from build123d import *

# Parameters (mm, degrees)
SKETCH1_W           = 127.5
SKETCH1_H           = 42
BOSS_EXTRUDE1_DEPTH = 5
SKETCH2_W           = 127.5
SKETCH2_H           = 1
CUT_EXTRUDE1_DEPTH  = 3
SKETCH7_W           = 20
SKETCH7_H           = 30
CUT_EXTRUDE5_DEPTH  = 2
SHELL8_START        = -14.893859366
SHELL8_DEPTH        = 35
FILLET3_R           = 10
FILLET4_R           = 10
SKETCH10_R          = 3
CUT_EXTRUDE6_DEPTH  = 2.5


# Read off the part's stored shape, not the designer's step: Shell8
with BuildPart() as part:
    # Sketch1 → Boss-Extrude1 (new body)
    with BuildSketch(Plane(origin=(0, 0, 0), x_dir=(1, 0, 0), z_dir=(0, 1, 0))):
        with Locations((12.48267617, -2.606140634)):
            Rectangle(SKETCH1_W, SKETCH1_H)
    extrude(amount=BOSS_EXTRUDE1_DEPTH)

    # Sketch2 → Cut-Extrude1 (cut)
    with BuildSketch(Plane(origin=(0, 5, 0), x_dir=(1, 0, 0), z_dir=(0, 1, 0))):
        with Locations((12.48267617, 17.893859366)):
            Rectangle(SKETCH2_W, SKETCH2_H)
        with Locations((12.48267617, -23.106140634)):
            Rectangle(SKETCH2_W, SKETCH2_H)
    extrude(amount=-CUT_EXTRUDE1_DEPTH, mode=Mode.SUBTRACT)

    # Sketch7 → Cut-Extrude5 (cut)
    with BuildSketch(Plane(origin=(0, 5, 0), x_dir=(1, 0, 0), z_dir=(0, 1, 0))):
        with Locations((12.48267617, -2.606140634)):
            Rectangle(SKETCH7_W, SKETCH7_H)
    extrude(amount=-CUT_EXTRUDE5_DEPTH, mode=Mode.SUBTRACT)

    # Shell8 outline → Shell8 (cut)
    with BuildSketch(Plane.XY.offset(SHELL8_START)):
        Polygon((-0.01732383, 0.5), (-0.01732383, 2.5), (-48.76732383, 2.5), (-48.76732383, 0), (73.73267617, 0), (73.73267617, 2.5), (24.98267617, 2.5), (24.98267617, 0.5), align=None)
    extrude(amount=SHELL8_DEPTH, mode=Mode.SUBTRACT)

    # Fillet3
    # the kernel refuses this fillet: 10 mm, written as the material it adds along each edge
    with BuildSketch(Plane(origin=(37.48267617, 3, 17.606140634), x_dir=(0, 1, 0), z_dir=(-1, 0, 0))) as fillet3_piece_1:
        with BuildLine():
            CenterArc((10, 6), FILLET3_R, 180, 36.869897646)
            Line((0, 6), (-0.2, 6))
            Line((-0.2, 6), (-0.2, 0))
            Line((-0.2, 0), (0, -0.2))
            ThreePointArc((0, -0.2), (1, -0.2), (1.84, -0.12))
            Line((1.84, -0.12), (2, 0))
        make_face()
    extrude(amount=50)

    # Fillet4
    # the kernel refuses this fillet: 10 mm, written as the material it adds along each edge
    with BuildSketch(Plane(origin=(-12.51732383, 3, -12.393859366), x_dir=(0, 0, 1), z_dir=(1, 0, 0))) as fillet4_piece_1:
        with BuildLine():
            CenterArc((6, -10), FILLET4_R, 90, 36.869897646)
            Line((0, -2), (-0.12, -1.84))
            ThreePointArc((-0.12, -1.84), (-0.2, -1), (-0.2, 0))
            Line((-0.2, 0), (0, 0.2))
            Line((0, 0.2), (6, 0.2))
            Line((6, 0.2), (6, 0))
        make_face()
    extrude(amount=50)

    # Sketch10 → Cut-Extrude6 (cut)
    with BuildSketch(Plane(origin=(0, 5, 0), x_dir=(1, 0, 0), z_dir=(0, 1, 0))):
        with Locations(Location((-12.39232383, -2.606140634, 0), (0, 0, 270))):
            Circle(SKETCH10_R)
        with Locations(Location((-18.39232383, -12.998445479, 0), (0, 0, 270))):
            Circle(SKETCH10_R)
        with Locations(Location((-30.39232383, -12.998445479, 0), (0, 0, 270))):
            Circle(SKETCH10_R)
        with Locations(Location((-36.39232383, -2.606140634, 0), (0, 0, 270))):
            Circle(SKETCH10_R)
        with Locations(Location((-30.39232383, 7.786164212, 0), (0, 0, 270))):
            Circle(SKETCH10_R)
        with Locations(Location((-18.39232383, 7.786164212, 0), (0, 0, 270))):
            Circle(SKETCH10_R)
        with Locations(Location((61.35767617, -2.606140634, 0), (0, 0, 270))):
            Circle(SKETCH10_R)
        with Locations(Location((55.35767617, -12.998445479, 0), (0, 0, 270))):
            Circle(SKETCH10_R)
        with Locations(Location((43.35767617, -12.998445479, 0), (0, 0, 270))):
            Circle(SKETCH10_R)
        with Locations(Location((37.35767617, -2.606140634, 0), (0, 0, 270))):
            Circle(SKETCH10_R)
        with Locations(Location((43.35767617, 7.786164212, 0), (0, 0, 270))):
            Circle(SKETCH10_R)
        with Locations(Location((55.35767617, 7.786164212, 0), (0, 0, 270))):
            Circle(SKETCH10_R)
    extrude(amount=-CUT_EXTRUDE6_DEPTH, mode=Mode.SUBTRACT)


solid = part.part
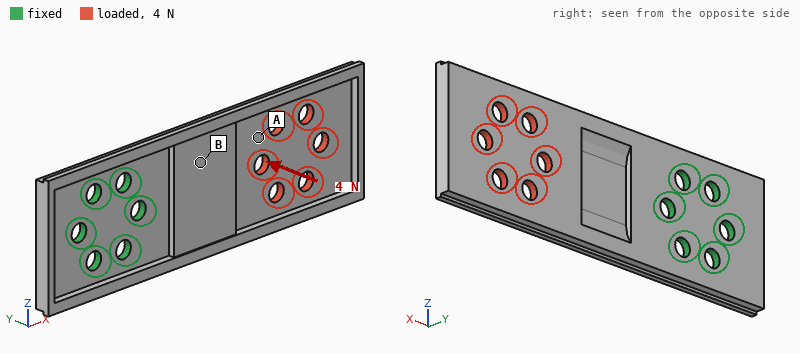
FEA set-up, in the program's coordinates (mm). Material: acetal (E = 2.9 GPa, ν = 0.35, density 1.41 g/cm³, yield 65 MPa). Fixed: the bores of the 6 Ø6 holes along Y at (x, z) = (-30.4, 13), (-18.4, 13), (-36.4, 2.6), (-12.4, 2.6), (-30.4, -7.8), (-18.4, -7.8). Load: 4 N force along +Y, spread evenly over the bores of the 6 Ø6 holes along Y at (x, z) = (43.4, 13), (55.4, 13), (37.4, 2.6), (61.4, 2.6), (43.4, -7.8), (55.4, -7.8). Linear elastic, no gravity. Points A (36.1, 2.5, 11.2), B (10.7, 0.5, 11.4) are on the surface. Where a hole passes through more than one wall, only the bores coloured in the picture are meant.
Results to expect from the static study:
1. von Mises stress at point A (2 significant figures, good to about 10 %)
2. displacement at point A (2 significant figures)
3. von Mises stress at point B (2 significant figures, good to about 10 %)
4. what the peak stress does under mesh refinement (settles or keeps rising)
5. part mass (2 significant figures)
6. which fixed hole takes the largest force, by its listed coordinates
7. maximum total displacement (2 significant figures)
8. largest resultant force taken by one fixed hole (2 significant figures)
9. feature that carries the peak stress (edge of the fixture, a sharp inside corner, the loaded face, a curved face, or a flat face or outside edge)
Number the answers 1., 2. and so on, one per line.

1. 0.49 MPa
2. 0.57 mm
3. 1.2 MPa
4. keeps rising
5. 21 g
6. (-12.4, 2.6)
7. 1.3 mm
8. 14 N
9. edge of the fixture
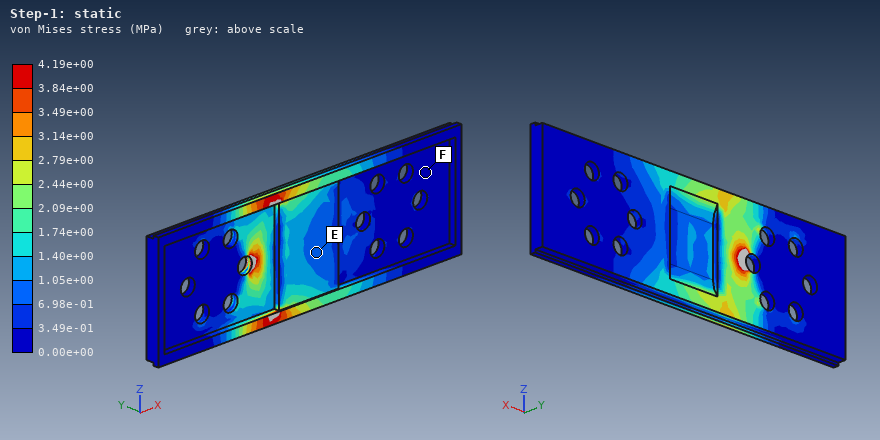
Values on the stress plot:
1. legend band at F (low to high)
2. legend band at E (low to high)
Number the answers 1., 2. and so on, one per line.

1. 0.00e+00 to 3.49e-01 MPa
2. 6.98e-01 to 1.05e+00 MPa
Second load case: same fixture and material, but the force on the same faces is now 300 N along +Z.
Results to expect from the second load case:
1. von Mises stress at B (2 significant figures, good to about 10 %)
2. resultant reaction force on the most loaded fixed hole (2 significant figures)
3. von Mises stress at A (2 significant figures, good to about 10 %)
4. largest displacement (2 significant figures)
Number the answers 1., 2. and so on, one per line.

1. 2.8 MPa
2. 450 N
3. 9.9 MPa
4. 1.4 mm
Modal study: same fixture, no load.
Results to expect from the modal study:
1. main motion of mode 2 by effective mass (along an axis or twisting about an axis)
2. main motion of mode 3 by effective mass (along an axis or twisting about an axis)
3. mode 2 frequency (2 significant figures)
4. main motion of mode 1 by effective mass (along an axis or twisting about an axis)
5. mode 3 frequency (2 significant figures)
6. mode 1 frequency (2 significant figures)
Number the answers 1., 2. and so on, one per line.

1. twisting about X
2. along Y
3. 350 Hz
4. along Y
5. 610 Hz
6. 110 Hz
